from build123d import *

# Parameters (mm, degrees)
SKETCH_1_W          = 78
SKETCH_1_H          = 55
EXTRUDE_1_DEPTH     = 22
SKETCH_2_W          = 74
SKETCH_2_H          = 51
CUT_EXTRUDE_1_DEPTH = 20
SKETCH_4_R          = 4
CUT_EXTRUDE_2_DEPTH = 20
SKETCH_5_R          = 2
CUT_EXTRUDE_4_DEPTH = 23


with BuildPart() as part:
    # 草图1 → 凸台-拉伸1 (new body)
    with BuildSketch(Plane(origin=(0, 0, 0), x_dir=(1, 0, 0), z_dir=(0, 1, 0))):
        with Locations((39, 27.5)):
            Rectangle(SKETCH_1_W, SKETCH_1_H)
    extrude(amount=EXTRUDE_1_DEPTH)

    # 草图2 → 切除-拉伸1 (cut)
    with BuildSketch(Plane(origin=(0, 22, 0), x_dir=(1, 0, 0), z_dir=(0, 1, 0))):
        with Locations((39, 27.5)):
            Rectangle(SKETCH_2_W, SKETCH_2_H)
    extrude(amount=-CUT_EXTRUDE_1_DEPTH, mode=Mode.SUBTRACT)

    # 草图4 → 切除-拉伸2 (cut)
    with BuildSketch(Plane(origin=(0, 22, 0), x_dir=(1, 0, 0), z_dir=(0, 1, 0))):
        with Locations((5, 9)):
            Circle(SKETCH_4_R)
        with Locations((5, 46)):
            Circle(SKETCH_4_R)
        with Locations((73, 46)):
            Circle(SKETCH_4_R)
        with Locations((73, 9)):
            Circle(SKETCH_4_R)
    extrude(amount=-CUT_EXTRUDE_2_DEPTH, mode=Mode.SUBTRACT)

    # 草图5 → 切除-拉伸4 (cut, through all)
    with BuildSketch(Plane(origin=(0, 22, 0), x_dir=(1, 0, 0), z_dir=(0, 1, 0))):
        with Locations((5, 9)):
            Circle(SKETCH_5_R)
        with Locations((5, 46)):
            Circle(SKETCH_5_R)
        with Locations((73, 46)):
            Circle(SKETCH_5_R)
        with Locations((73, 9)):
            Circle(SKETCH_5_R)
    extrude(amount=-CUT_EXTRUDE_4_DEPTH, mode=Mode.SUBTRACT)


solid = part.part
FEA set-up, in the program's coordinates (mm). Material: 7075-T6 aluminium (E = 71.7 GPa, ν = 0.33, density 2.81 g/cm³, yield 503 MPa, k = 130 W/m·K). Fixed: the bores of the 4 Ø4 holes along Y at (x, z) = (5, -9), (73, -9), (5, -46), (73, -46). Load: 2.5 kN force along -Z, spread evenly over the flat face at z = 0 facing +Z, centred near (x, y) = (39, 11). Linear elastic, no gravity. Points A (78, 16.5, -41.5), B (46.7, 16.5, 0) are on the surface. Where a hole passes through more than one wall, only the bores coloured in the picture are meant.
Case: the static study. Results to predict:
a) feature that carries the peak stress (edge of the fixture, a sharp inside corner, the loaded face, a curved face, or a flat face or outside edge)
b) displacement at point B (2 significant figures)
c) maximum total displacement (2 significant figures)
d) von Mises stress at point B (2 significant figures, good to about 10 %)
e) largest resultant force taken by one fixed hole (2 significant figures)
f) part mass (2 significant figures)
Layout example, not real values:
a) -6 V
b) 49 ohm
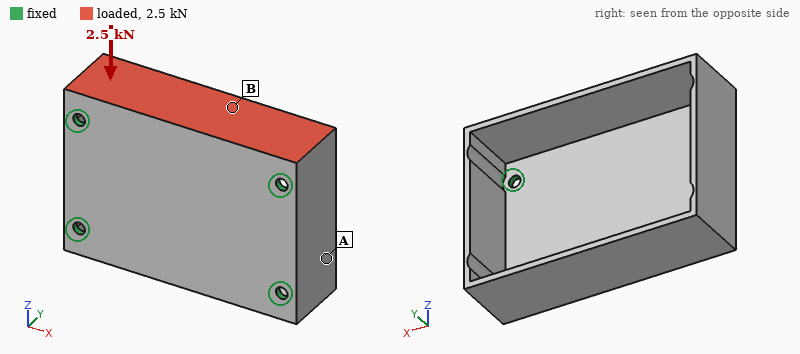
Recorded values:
a) a curved face
b) 0.71 mm
c) 1.0 mm
d) 99 MPa
e) 830 N
f) 52 g
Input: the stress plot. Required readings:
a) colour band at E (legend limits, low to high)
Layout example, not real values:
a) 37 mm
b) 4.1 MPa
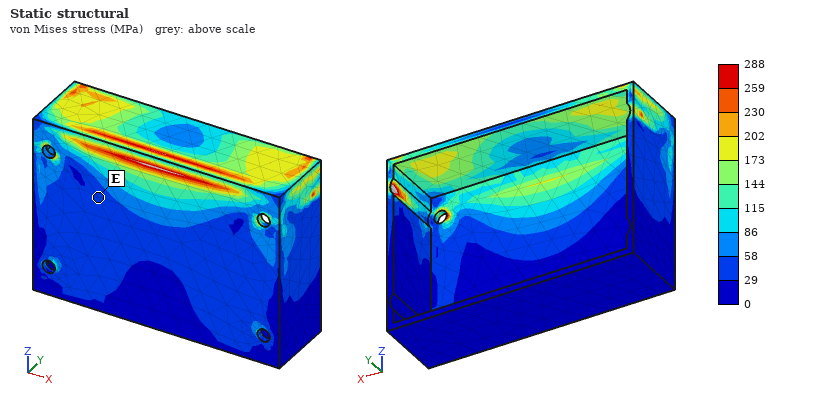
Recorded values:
a) 29 to 58 MPa
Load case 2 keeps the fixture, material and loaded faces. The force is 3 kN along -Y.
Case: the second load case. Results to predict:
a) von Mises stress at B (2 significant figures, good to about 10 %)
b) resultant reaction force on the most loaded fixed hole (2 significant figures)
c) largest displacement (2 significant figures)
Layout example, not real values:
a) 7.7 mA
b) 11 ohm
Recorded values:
a) 47 MPa
b) 2.0 kN
c) 0.29 mm
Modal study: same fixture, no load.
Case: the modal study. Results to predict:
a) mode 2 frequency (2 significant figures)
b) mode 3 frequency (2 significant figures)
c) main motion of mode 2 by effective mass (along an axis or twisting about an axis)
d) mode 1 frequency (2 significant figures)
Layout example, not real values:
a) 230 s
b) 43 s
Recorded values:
a) 3500 Hz
b) 4300 Hz
c) along Z
d) 2900 Hz
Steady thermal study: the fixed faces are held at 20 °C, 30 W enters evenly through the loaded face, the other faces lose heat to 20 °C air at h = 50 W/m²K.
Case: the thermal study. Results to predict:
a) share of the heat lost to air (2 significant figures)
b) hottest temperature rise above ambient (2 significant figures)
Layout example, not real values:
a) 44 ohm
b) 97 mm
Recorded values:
a) 22 %
b) 32 K
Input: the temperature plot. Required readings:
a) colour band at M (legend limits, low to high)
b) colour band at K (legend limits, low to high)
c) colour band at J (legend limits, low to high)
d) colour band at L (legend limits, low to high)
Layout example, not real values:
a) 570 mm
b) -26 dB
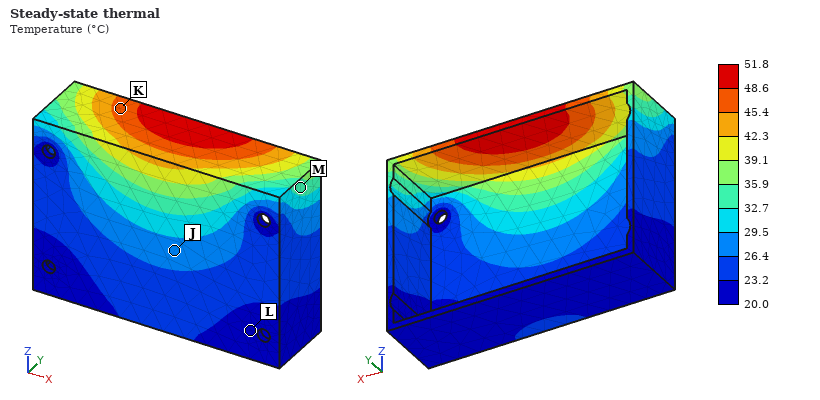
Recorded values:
a) 32.7 to 35.9 °C
b) 45.4 to 48.6 °C
c) 26.4 to 29.5 °C
d) 20.0 to 23.2 °C
